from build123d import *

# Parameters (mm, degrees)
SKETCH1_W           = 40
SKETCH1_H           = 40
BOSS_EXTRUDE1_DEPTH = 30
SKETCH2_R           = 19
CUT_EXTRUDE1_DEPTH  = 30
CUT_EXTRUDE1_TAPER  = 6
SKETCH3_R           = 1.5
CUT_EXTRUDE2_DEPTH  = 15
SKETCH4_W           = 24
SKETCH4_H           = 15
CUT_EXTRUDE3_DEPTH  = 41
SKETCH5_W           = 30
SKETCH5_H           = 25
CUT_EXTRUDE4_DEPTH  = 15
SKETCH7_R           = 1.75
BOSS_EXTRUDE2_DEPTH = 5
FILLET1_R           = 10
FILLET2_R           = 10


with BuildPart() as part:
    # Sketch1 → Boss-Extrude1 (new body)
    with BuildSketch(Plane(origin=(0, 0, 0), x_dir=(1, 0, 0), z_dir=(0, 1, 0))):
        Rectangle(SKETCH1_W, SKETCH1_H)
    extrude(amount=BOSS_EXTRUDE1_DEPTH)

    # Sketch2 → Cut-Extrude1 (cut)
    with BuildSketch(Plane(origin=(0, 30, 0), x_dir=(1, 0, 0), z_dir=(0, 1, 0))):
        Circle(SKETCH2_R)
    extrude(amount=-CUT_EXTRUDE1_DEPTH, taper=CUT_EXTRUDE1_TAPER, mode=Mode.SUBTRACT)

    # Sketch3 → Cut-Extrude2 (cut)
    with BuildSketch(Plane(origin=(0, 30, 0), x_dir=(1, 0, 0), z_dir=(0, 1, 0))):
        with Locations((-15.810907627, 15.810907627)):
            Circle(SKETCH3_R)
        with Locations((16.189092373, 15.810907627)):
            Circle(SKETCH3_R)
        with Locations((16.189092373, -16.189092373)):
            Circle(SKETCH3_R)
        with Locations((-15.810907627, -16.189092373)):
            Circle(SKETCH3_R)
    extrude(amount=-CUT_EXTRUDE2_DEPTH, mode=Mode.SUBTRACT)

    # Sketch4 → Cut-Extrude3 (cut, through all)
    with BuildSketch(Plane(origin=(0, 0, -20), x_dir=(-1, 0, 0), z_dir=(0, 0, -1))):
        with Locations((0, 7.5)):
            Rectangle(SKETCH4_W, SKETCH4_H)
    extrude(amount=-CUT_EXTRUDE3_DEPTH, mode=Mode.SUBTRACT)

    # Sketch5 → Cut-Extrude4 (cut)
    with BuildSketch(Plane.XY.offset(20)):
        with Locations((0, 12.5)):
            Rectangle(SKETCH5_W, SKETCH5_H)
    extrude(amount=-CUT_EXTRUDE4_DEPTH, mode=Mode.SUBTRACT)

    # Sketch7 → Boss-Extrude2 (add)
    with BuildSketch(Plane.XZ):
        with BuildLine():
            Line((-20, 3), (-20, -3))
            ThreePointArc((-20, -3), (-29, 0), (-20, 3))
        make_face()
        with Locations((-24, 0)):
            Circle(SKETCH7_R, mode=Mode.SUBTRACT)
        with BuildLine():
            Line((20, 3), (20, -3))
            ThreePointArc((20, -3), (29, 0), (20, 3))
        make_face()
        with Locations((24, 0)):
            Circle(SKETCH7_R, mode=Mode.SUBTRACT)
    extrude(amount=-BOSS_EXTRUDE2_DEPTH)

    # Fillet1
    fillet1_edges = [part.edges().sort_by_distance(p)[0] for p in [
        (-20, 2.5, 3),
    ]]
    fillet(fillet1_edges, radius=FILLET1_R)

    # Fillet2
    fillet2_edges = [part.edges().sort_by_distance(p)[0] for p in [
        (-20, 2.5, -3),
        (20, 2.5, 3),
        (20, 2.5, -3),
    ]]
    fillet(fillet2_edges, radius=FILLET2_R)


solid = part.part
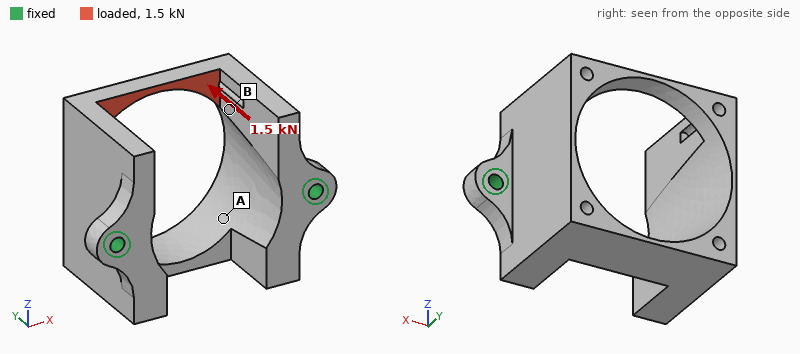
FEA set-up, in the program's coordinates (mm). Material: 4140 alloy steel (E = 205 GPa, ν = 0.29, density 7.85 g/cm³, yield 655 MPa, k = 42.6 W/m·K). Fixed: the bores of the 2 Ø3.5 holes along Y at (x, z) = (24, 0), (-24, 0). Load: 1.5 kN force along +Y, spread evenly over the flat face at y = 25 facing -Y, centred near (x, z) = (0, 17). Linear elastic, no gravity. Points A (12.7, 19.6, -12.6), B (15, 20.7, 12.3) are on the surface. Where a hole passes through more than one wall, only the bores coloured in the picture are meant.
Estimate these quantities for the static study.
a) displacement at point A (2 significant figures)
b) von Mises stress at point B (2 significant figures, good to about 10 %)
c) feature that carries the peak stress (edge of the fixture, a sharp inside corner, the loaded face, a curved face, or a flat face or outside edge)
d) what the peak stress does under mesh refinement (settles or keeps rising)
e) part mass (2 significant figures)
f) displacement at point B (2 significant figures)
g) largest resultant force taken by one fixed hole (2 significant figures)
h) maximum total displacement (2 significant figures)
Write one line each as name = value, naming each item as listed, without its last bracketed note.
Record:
displacement at point A = 0.034 mm
von Mises stress at point B = 78 MPa
feature that carries the peak stress = edge of the fixture
what the peak stress does under mesh refinement = keeps rising
part mass = 110 g
displacement at point B = 0.044 mm
largest resultant force taken by one fixed hole = 800 N
maximum total displacement = 0.11 mm
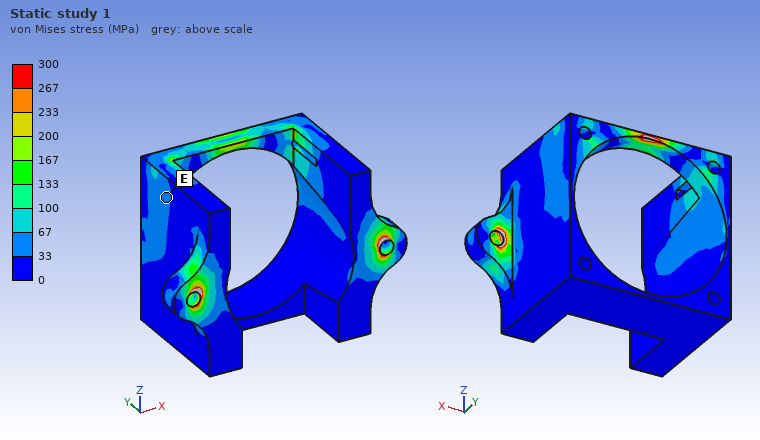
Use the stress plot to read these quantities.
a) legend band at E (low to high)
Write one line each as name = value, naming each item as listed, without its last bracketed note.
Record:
legend band at E = 33 to 67 MPa
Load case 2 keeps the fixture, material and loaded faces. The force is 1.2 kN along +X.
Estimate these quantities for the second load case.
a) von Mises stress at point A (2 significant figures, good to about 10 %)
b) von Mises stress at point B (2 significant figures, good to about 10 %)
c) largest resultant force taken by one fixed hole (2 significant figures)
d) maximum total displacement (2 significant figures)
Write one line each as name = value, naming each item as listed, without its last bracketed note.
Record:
von Mises stress at point A = 27 MPa
von Mises stress at point B = 41 MPa
largest resultant force taken by one fixed hole = 730 N
maximum total displacement = 0.12 mm
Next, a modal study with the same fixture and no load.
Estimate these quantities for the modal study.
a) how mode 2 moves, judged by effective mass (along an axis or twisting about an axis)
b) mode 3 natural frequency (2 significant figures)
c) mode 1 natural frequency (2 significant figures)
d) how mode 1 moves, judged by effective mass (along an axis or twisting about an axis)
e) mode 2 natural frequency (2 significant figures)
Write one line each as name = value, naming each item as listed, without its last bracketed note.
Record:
how mode 2 moves, judged by effective mass = along X
mode 3 natural frequency = 5200 Hz
mode 1 natural frequency = 2900 Hz
how mode 1 moves, judged by effective mass = along Z
mode 2 natural frequency = 4000 Hz
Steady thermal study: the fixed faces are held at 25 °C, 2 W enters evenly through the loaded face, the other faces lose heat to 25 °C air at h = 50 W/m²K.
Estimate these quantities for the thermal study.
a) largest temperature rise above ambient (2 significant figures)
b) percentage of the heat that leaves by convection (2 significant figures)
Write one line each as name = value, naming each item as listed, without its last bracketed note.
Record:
largest temperature rise above ambient = 14 K
percentage of the heat that leaves by convection = 50 %
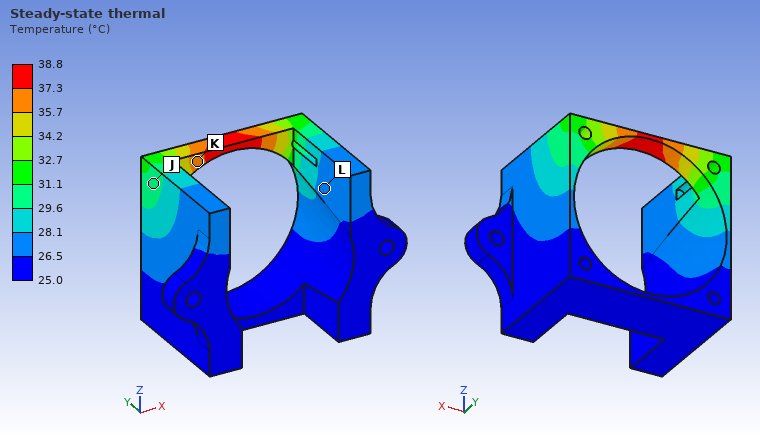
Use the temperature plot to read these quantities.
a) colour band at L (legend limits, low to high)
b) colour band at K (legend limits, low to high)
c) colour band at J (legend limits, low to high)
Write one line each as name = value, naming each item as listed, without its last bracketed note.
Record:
colour band at L = 26.5 to 28.1 °C
colour band at K = 35.7 to 37.3 °C
colour band at J = 29.6 to 31.1 °C
